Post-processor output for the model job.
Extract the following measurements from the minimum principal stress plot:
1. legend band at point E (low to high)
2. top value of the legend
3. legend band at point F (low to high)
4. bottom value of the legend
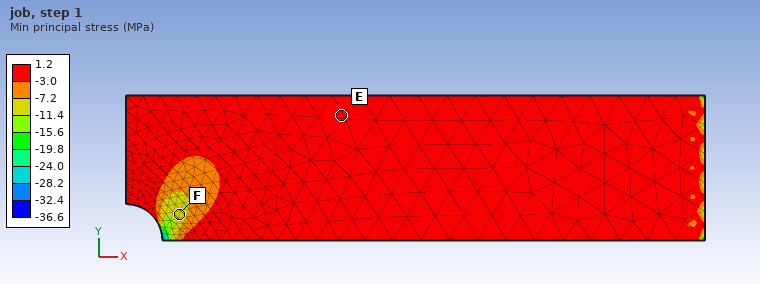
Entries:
-3.0 to 1.2 MPa
1.2 MPa
-11.4 to -7.2 MPa
-36.6 MPa
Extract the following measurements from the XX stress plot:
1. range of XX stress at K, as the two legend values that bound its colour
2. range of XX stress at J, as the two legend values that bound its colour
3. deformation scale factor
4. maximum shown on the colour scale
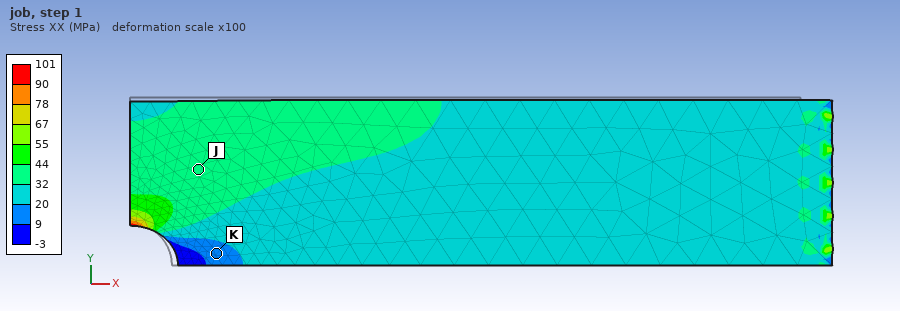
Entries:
9 to 20 MPa
32 to 44 MPa
100
101 MPa
